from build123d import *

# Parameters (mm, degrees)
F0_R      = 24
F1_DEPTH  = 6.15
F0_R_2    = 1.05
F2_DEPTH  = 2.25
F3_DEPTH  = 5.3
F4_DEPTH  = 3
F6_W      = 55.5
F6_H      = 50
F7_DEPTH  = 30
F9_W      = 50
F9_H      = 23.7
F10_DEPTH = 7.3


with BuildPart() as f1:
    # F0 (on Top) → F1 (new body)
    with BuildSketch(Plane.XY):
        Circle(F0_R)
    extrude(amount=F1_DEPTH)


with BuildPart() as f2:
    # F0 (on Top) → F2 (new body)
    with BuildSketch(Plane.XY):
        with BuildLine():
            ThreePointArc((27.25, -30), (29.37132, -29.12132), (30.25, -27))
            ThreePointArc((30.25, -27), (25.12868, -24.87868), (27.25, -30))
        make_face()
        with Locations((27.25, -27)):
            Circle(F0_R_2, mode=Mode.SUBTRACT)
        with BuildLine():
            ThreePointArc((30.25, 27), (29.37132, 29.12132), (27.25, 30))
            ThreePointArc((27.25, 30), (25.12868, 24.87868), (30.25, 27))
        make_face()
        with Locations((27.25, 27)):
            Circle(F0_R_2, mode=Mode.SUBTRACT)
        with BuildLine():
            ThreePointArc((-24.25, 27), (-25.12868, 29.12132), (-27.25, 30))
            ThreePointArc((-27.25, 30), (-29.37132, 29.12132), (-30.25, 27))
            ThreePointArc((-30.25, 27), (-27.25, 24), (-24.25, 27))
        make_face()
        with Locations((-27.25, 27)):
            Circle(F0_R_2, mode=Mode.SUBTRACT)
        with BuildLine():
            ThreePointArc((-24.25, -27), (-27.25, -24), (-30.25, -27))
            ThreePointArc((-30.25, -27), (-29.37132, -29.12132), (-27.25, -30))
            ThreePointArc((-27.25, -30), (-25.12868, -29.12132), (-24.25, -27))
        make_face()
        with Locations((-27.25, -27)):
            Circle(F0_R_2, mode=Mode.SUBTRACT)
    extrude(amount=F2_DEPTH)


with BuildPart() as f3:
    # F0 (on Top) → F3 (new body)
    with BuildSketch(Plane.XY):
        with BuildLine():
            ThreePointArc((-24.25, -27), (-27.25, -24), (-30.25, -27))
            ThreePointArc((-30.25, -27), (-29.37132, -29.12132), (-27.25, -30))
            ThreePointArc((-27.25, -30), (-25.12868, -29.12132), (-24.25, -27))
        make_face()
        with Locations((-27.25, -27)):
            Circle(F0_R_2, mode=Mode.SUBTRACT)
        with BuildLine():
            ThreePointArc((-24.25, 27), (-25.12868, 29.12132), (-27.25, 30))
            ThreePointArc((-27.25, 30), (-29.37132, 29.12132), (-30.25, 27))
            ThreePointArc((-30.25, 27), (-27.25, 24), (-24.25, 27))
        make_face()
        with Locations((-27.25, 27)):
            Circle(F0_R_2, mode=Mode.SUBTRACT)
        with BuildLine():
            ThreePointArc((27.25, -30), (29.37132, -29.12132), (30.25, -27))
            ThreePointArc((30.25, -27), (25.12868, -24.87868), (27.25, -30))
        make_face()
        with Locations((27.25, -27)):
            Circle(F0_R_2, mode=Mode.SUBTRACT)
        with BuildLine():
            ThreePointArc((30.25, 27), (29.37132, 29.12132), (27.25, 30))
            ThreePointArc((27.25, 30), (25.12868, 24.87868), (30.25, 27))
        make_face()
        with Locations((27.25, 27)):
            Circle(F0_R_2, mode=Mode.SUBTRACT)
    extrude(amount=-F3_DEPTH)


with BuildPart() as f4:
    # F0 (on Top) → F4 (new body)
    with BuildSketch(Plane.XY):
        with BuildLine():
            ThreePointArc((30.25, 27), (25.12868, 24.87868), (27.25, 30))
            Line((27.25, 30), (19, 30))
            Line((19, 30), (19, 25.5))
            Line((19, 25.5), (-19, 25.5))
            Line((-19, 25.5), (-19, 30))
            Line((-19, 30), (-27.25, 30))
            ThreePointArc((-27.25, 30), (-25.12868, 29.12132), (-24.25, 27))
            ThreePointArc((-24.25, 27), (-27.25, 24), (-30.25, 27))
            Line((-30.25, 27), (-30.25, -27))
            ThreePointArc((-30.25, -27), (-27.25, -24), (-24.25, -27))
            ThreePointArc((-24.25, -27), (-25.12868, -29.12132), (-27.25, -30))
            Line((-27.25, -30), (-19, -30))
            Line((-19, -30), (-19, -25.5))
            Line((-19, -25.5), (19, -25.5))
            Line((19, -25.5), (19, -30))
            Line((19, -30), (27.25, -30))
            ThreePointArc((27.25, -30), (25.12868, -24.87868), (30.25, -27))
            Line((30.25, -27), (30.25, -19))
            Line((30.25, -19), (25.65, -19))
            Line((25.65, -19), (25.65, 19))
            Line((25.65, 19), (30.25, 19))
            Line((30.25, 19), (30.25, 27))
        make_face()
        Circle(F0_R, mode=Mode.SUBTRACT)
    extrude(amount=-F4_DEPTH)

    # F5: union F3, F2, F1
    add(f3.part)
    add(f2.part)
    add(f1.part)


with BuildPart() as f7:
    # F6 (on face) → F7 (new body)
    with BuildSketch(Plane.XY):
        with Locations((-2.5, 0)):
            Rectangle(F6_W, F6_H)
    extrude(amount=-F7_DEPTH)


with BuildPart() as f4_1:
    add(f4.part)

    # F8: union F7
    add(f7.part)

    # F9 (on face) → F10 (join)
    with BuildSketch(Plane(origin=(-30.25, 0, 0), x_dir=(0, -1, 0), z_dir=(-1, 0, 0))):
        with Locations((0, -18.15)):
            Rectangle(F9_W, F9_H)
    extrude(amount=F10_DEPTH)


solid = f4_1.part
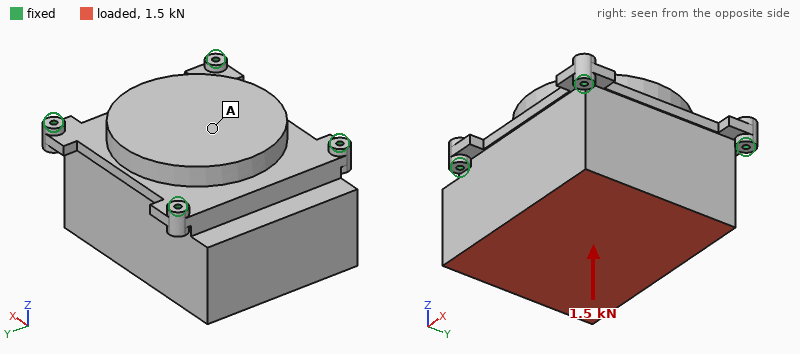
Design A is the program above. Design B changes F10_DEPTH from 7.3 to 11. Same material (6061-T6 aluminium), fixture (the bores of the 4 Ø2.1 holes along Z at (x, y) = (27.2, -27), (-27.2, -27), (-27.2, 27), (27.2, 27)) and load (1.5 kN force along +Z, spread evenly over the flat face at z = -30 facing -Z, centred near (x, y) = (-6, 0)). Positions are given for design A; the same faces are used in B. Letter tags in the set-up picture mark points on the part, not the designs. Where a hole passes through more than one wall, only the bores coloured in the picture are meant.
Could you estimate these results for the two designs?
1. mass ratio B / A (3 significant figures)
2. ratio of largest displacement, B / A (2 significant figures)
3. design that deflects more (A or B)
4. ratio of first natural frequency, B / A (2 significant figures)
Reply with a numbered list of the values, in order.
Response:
1. 1.04
2. 0.91
3. A
4. 0.99
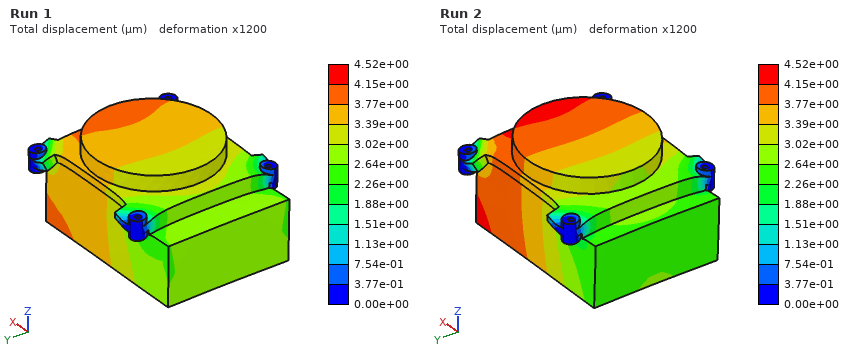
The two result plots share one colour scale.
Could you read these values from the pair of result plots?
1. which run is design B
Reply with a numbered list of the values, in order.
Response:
1. Run 1
